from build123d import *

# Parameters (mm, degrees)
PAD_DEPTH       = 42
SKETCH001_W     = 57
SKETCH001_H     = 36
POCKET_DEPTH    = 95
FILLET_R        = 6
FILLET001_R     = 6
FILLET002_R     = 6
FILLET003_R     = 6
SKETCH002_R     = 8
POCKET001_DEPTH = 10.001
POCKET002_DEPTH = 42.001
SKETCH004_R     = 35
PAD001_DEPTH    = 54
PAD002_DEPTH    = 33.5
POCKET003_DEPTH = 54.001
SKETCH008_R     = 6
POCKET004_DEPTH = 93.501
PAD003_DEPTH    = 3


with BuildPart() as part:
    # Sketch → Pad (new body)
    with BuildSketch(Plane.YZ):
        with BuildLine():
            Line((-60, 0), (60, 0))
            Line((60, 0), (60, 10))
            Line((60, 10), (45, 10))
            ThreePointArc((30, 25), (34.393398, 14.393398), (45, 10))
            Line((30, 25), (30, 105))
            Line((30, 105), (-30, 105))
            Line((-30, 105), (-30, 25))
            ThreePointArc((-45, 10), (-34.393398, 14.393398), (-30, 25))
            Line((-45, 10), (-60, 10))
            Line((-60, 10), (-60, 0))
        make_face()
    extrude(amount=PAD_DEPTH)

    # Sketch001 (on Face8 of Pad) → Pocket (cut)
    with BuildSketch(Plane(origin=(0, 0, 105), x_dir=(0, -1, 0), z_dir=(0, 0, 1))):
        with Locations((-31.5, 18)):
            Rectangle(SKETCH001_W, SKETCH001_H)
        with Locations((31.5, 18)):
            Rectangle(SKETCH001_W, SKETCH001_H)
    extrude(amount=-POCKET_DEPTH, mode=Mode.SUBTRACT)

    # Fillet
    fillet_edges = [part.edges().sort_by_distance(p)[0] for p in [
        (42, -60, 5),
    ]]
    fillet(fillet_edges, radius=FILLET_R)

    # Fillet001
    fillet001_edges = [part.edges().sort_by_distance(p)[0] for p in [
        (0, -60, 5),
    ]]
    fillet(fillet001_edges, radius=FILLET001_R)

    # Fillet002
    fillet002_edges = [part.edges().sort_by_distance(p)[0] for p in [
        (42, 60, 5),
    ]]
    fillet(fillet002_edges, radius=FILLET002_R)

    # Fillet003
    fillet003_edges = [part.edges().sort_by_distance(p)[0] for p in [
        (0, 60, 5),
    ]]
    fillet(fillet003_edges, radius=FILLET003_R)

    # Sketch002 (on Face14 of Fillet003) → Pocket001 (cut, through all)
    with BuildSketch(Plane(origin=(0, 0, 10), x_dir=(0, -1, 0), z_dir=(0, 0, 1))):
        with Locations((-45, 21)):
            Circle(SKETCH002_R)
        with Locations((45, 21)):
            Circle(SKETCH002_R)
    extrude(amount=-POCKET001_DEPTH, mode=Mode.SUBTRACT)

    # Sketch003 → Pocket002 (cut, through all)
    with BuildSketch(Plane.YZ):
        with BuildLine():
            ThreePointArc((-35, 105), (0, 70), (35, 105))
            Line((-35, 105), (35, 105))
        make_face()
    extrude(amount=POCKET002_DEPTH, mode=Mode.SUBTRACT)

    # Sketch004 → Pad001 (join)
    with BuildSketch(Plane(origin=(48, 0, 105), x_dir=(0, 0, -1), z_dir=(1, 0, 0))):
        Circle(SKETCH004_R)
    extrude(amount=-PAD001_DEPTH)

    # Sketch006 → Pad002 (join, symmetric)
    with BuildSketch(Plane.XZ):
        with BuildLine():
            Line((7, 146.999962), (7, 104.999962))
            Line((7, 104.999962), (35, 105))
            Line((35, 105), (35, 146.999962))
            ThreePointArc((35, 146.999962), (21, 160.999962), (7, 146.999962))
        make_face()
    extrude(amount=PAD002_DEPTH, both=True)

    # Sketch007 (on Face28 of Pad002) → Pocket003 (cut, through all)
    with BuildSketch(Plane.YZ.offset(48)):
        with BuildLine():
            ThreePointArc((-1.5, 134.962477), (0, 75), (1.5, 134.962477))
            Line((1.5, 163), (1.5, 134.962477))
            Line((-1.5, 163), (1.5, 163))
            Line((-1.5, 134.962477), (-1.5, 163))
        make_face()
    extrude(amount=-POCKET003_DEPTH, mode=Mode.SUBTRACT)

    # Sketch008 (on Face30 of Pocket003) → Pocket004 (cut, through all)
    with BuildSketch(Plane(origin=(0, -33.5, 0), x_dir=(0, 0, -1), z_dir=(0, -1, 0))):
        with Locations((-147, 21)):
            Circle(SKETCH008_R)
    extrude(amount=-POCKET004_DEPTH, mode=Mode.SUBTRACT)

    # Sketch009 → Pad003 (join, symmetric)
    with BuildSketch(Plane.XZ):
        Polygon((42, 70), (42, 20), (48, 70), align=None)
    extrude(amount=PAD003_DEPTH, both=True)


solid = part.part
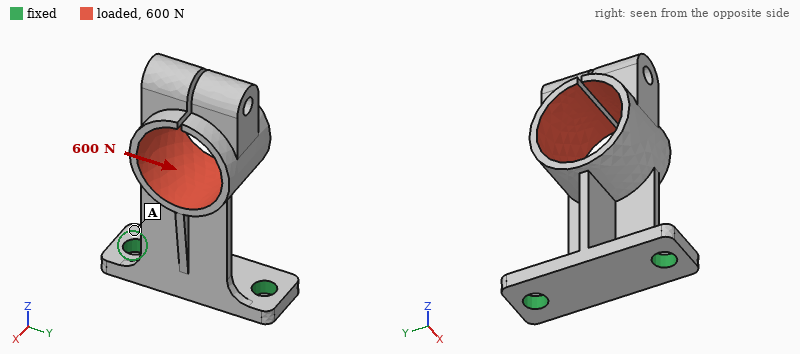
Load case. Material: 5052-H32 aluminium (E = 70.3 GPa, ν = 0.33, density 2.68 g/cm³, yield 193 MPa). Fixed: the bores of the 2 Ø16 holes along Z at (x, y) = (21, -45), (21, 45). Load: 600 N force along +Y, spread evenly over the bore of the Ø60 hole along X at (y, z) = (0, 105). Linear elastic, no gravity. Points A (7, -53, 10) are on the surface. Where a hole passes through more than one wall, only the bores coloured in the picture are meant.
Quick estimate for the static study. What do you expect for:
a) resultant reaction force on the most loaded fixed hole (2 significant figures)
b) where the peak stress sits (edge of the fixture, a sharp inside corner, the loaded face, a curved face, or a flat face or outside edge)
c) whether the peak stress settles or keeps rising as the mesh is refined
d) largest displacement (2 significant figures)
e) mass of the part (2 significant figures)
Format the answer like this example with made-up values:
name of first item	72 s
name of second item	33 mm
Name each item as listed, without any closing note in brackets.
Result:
resultant reaction force on the most loaded fixed hole	900 N
where the peak stress sits	a sharp inside corner
whether the peak stress settles or keeps rising as the mesh is refined	keeps rising
largest displacement	0.51 mm
mass of the part	470 g
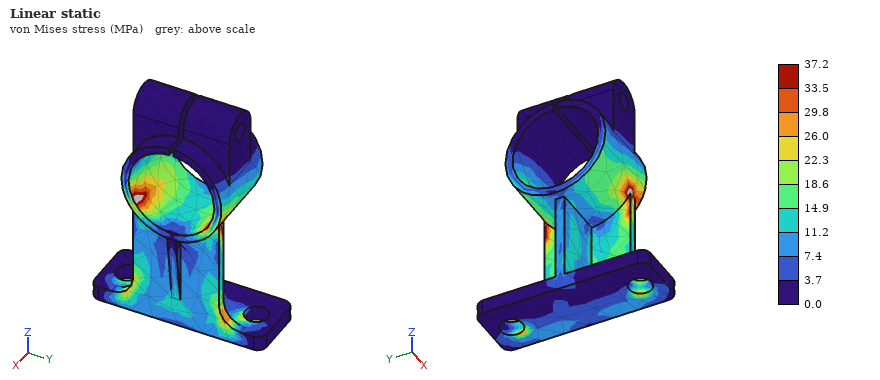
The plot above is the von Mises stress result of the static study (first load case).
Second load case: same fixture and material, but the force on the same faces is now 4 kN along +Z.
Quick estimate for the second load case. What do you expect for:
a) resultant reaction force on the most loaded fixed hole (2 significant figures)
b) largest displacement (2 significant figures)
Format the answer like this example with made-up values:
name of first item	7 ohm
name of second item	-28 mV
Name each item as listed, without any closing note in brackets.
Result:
resultant reaction force on the most loaded fixed hole	2.1 kN
largest displacement	0.68 mm
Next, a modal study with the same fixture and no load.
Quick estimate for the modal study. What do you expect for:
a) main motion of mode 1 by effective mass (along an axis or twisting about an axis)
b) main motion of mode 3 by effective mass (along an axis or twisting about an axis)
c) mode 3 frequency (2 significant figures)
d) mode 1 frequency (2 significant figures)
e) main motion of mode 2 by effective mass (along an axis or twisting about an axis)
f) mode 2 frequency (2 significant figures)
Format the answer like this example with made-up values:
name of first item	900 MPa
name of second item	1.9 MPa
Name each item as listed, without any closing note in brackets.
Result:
main motion of mode 1 by effective mass	along Y
main motion of mode 3 by effective mass	along X
mode 3 frequency	410 Hz
mode 1 frequency	320 Hz
main motion of mode 2 by effective mass	along X
mode 2 frequency	340 Hz
